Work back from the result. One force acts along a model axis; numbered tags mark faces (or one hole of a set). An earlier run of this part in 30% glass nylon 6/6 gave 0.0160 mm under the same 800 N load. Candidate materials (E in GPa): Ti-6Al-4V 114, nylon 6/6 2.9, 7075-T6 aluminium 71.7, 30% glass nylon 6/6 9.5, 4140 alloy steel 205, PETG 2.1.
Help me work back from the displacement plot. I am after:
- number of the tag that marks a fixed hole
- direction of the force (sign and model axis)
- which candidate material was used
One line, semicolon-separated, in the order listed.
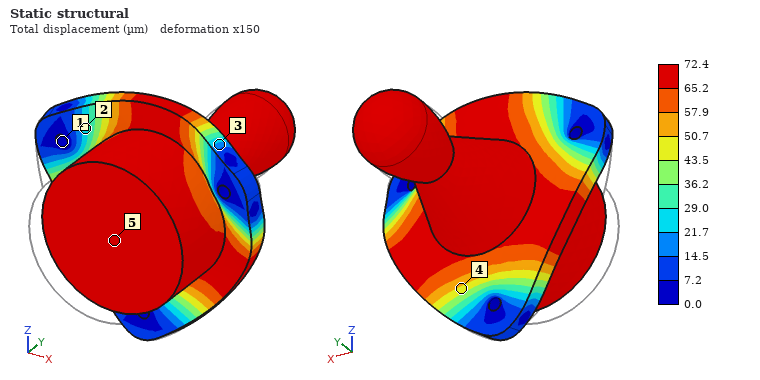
1; +Y; PETG
